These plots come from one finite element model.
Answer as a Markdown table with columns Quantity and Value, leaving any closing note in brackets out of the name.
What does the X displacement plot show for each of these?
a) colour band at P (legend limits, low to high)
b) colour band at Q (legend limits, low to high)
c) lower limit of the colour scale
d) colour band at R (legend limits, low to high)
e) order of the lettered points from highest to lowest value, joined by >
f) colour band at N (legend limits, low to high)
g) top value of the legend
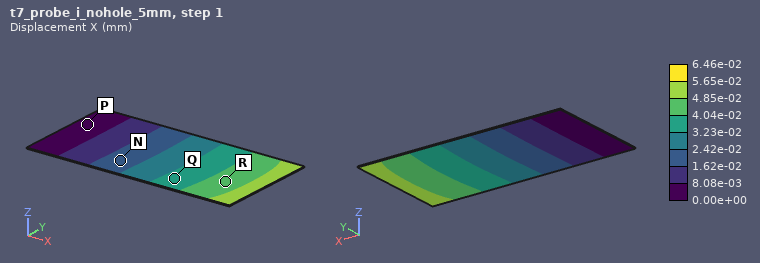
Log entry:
| Quantity | Value |
|---|---|
| colour band at P | 0.00e+00 to 8.08e-03 mm |
| colour band at Q | 3.23e-02 to 4.04e-02 mm |
| lower limit of the colour scale | 0.00e+00 mm |
| colour band at R | 4.04e-02 to 4.85e-02 mm |
| order of the lettered points from highest to lowest value, joined by > | R > Q > N > P |
| colour band at N | 1.62e-02 to 2.42e-02 mm |
| top value of the legend | 6.46e-02 mm |
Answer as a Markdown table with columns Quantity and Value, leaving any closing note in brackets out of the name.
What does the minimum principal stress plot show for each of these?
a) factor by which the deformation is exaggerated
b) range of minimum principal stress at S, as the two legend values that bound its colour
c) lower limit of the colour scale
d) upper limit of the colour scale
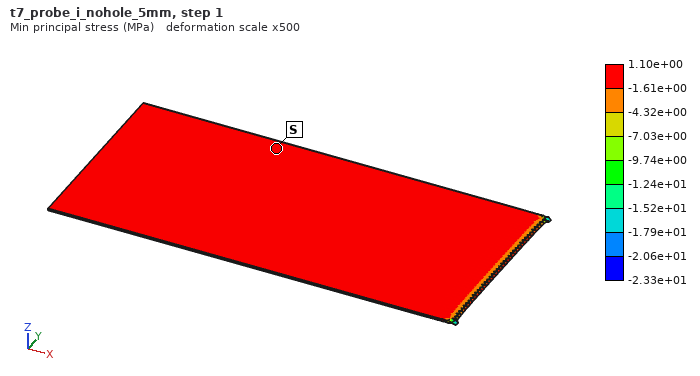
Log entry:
| Quantity | Value |
|---|---|
| factor by which the deformation is exaggerated | 500 |
| range of minimum principal stress at S, as the two legend values that bound its colour | -1.61e+00 to 1.10e+00 MPa |
| lower limit of the colour scale | -2.33e+01 MPa |
| upper limit of the colour scale | 1.10e+00 MPa |
